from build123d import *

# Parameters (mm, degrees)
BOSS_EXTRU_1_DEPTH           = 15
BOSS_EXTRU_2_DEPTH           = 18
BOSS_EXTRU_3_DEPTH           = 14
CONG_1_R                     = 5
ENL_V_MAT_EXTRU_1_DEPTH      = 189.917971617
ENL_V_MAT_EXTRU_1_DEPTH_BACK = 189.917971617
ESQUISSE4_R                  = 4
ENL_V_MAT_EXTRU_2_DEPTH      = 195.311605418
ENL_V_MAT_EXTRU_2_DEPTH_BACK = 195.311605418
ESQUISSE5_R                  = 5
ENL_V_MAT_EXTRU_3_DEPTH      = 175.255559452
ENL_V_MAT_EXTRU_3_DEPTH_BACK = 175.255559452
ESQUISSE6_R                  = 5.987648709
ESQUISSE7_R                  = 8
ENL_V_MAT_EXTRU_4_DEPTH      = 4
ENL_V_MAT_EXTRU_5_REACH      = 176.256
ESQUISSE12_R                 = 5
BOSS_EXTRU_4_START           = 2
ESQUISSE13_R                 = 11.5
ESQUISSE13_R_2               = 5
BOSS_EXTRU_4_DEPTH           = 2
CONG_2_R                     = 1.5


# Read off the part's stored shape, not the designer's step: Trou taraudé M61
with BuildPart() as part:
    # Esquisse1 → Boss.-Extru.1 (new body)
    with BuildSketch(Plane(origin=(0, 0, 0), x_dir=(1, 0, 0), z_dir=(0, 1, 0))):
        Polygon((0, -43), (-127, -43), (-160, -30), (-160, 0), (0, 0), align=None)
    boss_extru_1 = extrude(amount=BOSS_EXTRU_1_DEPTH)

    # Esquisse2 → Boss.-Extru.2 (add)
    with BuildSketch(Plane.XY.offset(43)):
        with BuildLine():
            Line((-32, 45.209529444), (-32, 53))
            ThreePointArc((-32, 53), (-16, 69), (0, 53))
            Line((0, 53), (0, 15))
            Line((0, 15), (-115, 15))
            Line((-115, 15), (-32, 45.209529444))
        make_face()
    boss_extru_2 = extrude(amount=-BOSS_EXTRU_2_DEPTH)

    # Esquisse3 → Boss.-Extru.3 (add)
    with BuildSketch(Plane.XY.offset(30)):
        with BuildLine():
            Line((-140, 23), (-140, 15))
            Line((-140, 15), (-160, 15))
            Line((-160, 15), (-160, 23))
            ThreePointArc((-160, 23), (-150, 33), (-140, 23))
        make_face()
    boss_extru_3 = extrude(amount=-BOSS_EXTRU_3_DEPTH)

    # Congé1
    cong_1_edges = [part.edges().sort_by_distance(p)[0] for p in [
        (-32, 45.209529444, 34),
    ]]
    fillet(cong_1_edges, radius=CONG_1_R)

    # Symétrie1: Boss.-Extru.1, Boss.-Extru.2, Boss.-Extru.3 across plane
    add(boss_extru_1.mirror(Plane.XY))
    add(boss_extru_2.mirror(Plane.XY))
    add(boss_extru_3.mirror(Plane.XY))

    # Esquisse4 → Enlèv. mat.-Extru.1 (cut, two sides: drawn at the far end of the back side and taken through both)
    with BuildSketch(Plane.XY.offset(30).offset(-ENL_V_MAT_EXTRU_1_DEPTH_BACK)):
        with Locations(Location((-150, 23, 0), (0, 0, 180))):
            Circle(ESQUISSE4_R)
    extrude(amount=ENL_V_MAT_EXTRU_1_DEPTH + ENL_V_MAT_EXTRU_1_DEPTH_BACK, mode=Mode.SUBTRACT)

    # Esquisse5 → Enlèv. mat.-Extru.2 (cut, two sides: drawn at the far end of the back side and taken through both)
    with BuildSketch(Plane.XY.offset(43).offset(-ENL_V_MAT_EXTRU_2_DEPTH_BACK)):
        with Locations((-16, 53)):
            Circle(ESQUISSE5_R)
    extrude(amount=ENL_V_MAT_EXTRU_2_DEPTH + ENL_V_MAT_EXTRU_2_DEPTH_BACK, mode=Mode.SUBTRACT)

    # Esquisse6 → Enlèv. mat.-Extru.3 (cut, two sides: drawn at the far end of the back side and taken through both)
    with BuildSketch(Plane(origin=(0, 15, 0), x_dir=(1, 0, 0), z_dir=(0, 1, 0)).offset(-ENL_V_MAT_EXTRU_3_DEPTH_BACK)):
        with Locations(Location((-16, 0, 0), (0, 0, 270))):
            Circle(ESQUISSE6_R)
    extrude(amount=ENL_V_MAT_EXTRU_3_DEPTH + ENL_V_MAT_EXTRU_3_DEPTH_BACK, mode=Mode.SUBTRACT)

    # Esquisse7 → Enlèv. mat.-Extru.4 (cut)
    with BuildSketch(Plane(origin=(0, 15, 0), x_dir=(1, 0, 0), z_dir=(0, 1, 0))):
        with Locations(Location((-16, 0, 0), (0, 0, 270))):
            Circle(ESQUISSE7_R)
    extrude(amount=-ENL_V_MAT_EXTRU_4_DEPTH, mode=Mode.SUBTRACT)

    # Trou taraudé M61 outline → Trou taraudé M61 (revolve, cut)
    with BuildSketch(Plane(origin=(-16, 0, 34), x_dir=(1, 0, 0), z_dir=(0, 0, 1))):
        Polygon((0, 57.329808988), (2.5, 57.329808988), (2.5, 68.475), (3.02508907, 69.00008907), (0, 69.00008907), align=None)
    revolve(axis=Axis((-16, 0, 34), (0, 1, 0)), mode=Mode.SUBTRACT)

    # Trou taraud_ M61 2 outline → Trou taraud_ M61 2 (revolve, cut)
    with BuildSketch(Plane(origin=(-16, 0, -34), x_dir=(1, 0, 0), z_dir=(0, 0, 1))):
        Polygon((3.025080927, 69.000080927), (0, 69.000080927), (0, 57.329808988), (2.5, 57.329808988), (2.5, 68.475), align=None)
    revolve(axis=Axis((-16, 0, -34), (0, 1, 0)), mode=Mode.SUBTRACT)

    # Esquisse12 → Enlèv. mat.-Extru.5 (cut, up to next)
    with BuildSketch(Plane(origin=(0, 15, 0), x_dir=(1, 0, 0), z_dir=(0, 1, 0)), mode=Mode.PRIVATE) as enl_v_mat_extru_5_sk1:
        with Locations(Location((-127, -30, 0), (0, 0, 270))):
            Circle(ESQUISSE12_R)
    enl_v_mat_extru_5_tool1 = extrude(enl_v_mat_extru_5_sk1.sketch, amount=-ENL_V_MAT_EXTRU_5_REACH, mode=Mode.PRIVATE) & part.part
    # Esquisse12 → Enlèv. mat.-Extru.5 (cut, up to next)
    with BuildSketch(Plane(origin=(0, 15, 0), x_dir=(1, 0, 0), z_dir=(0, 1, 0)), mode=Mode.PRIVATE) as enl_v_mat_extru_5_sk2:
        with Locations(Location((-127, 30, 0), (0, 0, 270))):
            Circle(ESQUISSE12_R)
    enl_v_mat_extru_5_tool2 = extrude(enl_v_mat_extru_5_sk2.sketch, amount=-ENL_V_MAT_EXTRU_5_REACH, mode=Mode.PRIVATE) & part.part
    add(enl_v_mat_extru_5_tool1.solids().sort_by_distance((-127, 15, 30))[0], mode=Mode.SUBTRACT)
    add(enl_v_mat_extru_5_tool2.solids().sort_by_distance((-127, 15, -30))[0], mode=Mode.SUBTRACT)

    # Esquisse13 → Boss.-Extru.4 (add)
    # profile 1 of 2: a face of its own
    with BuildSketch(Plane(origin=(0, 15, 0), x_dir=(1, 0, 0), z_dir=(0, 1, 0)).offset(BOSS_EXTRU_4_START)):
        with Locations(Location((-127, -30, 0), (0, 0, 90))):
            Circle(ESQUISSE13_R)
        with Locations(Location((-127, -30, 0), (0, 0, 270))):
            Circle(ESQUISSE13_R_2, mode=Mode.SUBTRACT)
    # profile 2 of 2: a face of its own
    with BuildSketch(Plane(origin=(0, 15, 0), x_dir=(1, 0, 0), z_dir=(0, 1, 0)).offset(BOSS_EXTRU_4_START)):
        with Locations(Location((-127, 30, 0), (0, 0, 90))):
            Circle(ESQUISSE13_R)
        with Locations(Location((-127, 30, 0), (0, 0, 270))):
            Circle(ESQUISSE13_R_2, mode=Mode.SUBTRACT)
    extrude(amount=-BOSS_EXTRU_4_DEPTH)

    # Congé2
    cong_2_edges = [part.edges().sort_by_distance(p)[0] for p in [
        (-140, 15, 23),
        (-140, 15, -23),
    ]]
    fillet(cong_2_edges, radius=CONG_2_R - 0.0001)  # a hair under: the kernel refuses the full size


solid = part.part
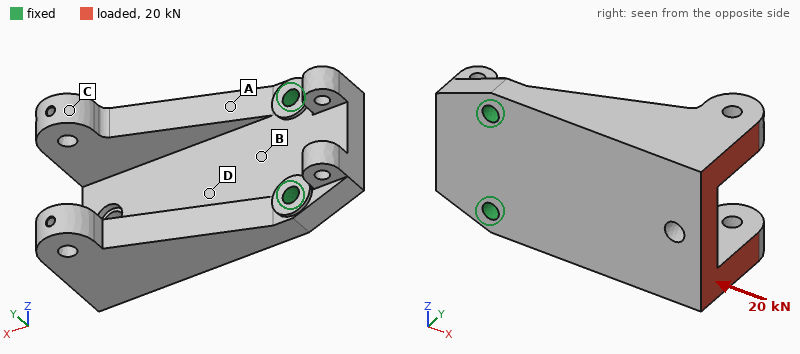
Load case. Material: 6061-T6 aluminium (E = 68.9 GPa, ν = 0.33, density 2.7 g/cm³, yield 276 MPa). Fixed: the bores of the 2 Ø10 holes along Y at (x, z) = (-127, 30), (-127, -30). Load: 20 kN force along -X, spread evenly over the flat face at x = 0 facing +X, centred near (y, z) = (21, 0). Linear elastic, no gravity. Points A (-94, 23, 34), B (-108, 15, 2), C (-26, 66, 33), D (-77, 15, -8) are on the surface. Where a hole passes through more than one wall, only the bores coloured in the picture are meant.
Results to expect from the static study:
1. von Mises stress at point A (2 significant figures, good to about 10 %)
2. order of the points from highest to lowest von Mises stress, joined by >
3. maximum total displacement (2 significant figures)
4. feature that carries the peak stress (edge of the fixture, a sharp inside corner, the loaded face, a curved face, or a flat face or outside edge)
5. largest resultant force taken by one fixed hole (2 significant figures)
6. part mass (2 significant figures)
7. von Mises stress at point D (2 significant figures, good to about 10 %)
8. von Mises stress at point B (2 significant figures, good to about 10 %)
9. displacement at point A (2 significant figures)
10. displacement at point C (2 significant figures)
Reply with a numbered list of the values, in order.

1. 64 MPa
2. A > B > D > C
3. 0.65 mm
4. a flat face or outside edge
5. 10 kN
6. 820 g
7. 27 MPa
8. 51 MPa
9. 0.11 mm
10. 0.55 mm
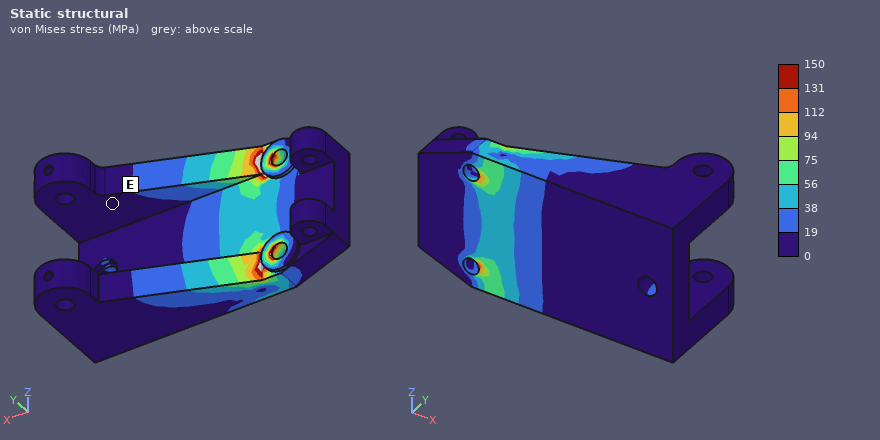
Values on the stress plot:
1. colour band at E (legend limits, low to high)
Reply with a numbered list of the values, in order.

1. 0 to 19 MPa
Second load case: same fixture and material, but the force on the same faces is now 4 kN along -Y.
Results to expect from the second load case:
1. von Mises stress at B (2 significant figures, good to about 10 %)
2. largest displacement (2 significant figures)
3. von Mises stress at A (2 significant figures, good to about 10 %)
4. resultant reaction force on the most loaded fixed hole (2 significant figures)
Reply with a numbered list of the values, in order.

1. 75 MPa
2. 1.1 mm
3. 80 MPa
4. 2.1 kN
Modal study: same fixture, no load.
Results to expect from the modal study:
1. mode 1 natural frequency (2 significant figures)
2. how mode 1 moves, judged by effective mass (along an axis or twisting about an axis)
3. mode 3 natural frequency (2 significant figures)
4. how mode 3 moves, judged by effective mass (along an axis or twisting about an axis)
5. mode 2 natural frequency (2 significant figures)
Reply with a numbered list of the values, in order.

1. 610 Hz
2. along Y
3. 2500 Hz
4. along Z
5. 1400 Hz
